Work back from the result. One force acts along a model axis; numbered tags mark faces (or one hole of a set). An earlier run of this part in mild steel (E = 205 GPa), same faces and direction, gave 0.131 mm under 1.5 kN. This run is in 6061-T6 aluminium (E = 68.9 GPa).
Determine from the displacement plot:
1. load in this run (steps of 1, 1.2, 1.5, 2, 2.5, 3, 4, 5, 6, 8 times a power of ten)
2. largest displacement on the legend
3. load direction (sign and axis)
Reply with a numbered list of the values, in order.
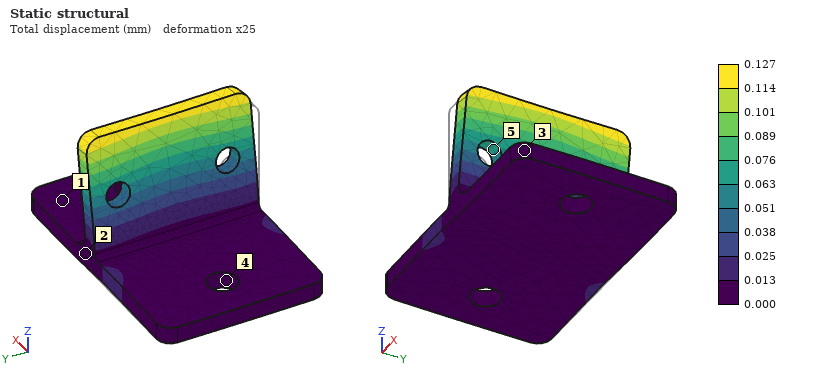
1. 500 N
2. 0.127 mm
3. +X
